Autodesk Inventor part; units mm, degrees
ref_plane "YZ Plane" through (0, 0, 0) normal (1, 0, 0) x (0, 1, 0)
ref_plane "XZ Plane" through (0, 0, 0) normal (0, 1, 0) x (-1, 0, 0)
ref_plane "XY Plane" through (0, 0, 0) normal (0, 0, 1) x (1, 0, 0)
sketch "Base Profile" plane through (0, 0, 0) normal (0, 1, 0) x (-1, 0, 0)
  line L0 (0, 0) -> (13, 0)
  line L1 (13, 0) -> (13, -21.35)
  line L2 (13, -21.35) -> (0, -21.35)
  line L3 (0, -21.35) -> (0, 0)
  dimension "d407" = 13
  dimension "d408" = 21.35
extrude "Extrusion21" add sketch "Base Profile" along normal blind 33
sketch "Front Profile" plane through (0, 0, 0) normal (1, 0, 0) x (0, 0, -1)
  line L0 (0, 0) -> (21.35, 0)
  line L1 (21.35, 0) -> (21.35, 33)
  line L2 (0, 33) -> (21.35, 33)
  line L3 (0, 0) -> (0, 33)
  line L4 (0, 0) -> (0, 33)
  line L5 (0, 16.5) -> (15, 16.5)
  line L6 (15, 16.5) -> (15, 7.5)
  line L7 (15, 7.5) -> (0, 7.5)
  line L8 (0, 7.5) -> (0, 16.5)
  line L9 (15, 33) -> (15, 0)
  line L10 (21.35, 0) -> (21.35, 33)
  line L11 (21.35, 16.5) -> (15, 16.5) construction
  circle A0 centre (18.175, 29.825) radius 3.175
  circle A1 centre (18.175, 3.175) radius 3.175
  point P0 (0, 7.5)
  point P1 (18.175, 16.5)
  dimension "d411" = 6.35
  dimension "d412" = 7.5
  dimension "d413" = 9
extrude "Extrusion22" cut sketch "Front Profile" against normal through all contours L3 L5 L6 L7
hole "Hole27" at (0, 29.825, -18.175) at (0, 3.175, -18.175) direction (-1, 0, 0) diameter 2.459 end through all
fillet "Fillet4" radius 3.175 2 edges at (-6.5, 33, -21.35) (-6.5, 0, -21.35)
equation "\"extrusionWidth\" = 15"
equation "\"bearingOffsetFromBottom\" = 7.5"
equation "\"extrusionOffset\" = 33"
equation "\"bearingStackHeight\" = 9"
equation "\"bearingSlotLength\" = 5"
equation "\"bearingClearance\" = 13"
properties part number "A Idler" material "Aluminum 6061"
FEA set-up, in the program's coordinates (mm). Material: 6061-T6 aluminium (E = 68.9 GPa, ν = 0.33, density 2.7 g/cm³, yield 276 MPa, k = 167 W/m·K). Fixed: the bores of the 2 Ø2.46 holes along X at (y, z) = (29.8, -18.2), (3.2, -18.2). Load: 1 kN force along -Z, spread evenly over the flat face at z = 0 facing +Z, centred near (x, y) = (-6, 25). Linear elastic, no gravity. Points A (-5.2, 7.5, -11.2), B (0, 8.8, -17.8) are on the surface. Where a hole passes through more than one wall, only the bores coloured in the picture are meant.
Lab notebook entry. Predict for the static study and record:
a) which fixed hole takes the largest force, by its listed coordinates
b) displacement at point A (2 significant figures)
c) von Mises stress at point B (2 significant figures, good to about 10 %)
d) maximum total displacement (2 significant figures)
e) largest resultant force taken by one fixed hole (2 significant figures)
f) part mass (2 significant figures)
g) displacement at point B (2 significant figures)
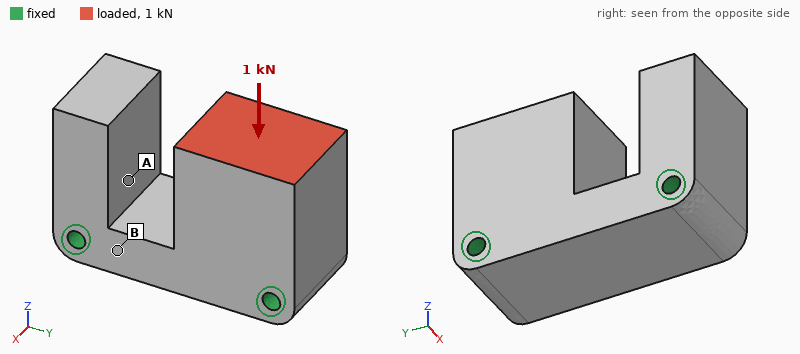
(29.8, -18.2)
1.5 µm
7.1 MPa
6.6 µm
820 N
20 g
1.4 µm
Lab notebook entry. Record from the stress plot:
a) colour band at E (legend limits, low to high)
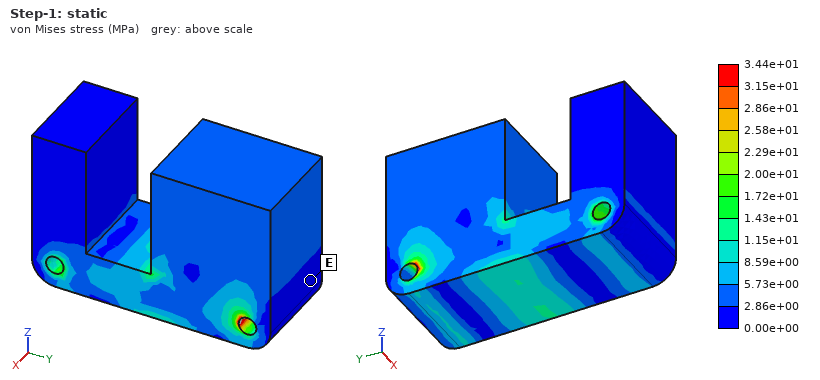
0.00e+00 to 2.86e+00 MPa
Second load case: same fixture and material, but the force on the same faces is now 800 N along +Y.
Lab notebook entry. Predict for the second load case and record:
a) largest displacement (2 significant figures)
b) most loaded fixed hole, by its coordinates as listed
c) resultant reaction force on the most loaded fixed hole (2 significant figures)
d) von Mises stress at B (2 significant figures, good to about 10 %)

22 µm
(29.8, -18.2)
720 N
20 MPa
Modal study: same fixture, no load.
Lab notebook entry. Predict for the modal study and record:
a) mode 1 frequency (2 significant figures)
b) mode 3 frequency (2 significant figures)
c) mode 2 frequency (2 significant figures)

13 kHz
18 kHz
18 kHz
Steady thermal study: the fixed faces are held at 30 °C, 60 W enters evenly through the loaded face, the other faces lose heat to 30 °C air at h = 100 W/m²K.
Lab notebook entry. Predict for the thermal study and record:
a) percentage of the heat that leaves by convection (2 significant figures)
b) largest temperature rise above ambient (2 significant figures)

4.0 %
34 K
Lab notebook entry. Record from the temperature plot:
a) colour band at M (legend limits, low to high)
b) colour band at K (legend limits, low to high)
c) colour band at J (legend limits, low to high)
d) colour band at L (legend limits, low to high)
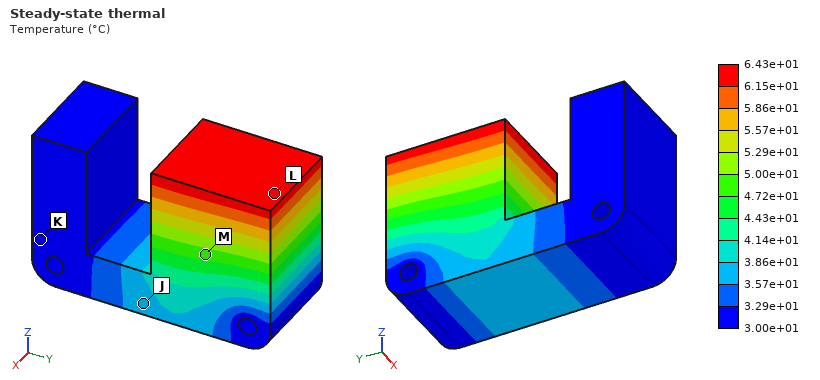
4.72e+01 to 5.00e+01 °C
3.00e+01 to 3.29e+01 °C
3.57e+01 to 3.86e+01 °C
6.15e+01 to 6.43e+01 °C
